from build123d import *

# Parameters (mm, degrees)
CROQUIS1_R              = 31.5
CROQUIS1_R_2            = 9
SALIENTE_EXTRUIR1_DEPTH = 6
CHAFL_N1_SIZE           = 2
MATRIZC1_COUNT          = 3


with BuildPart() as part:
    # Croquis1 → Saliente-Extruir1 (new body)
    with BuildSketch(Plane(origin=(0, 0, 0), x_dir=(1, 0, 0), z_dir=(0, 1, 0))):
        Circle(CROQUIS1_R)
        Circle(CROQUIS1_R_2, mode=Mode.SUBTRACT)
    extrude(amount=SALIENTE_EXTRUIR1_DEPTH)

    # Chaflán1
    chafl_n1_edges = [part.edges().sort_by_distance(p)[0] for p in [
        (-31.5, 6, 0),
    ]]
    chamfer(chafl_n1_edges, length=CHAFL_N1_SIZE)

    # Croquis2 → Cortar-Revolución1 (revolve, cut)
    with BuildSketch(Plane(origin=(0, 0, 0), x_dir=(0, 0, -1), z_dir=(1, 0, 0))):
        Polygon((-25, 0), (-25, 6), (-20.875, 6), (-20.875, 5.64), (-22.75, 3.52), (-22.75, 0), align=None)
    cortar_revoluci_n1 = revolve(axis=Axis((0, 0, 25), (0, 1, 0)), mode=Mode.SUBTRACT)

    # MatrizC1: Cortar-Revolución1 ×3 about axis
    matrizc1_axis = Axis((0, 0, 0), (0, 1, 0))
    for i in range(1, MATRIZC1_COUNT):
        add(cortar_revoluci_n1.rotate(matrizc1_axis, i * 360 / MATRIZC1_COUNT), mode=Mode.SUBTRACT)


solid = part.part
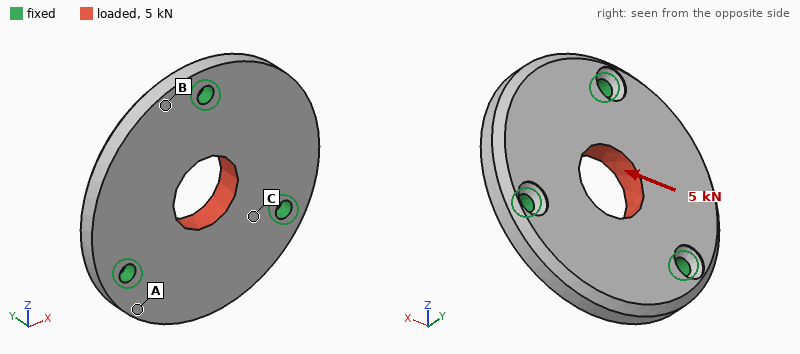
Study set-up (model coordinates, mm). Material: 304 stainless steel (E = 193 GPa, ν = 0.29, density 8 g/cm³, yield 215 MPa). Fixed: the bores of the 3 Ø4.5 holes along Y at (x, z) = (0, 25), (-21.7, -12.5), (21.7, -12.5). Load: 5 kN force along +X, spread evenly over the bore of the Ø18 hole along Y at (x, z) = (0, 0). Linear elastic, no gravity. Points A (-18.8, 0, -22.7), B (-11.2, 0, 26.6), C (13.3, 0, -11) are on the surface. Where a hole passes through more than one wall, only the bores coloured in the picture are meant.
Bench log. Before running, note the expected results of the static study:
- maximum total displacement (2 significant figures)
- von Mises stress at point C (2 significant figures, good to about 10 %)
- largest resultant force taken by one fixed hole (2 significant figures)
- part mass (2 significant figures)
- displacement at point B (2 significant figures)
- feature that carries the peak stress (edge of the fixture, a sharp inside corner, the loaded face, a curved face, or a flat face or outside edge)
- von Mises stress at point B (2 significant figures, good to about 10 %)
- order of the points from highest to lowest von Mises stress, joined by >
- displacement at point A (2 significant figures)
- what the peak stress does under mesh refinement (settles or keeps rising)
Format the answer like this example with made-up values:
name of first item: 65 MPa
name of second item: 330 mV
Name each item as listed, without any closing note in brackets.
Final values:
maximum total displacement: 3.2 µm
von Mises stress at point C: 22 MPa
largest resultant force taken by one fixed hole: 1.7 kN
part mass: 130 g
displacement at point B: 1.1 µm
feature that carries the peak stress: edge of the fixture
von Mises stress at point B: 11 MPa
order of the points from highest to lowest von Mises stress, joined by >: C > B > A
displacement at point A: 0.69 µm
what the peak stress does under mesh refinement: keeps rising
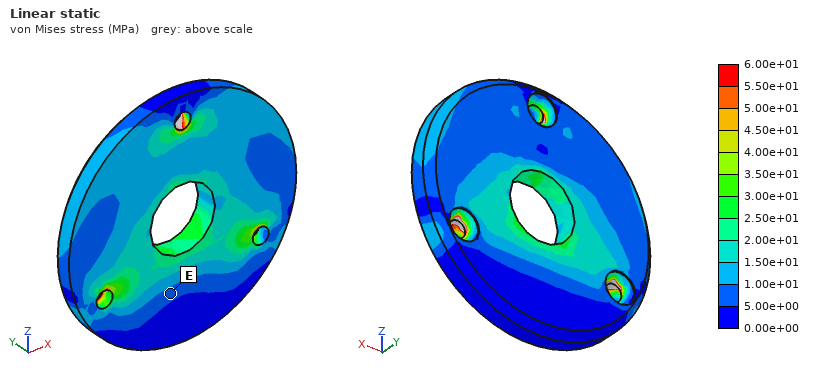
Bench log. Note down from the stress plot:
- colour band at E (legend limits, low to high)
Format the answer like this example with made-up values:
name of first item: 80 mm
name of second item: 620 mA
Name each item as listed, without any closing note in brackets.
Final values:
colour band at E: 5.00e+00 to 1.00e+01 MPa
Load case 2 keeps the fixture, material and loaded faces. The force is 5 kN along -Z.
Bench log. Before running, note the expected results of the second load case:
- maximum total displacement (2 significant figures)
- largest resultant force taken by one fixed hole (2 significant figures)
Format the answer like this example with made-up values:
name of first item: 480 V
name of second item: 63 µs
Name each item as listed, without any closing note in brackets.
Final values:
maximum total displacement: 3.4 µm
largest resultant force taken by one fixed hole: 1.7 kN
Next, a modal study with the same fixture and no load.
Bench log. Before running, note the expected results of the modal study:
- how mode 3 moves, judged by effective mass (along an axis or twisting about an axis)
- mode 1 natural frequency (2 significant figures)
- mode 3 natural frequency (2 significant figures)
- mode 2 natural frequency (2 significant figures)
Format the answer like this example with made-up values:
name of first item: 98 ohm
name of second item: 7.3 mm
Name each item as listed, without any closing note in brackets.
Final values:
how mode 3 moves, judged by effective mass: along Y
mode 1 natural frequency: 8000 Hz
mode 3 natural frequency: 9800 Hz
mode 2 natural frequency: 8000 Hz
